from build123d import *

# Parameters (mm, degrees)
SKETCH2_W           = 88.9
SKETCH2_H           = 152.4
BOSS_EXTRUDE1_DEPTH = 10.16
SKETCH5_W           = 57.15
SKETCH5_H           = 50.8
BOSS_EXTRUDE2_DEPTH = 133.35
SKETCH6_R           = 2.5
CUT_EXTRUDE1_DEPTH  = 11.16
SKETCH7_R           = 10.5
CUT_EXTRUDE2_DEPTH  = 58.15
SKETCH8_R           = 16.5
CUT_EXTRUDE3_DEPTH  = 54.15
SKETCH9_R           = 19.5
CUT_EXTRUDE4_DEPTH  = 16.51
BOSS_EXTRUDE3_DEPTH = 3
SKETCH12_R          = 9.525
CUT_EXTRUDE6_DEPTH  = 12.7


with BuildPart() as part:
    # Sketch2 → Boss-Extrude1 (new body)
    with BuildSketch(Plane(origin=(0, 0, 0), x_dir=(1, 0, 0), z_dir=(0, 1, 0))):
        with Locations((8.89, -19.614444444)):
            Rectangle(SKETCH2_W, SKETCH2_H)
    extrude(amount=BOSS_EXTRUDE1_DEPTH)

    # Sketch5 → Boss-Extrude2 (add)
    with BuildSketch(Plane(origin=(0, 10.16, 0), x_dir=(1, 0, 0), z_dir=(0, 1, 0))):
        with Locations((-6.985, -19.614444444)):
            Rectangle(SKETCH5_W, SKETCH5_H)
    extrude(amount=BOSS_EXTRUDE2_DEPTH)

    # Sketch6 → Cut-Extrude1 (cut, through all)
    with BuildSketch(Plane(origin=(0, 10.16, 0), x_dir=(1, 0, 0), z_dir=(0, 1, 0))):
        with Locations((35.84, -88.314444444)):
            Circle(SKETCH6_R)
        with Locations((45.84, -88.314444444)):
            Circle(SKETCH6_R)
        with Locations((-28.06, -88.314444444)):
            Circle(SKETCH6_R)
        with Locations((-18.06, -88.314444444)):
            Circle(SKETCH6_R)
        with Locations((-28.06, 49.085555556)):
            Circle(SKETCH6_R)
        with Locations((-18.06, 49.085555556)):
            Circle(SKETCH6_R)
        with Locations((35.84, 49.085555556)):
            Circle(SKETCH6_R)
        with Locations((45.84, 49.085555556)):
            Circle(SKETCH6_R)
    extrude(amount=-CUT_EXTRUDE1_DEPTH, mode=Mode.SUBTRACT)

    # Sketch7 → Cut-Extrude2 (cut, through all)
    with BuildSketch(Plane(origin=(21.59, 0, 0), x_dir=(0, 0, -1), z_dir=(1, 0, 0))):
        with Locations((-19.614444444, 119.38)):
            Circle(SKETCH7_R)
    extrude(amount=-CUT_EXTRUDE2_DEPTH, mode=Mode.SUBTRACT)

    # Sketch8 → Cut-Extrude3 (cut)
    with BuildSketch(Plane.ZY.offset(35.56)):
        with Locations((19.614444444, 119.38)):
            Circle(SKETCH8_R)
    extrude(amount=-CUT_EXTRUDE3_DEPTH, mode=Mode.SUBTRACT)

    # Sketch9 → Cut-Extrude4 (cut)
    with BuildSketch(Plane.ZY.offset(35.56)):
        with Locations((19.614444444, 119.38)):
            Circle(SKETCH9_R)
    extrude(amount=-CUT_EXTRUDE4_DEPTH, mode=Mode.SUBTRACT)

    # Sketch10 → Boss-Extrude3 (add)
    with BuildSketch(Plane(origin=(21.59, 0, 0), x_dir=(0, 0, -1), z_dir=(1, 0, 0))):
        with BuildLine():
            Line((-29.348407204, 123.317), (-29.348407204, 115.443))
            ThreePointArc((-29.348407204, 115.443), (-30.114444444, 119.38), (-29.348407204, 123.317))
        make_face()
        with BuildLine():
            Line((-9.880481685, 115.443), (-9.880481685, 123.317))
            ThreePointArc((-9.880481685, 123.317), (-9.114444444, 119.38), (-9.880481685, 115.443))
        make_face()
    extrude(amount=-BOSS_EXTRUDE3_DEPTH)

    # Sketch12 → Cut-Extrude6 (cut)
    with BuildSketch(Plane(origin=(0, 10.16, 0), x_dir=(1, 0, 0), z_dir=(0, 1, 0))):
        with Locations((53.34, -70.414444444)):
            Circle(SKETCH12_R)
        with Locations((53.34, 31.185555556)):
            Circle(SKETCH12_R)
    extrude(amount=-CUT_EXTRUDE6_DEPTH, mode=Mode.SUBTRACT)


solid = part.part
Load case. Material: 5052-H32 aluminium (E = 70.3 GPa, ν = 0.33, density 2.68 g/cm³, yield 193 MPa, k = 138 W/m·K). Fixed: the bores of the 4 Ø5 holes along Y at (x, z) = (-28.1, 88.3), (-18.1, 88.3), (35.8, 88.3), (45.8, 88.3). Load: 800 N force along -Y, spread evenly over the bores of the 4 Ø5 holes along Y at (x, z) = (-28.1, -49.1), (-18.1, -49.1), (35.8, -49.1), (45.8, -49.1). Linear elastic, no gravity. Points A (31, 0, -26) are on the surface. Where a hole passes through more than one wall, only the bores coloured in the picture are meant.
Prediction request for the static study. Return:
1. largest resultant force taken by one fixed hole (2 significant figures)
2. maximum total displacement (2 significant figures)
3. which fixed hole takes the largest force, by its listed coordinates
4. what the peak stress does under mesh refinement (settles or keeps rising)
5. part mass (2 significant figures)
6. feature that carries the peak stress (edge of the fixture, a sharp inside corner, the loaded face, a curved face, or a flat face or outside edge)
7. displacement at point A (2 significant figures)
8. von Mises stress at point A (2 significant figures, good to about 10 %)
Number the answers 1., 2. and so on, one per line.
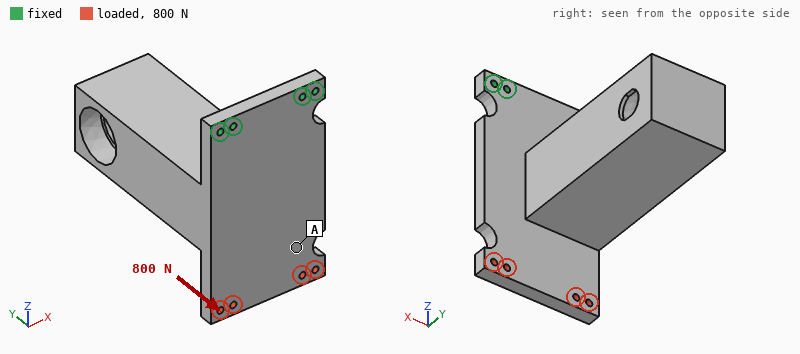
1. 390 N
2. 1.5 mm
3. (-18.1, 88.3)
4. keeps rising
5. 1.3 kg
6. edge of the fixture
7. 0.92 mm
8. 13 MPa
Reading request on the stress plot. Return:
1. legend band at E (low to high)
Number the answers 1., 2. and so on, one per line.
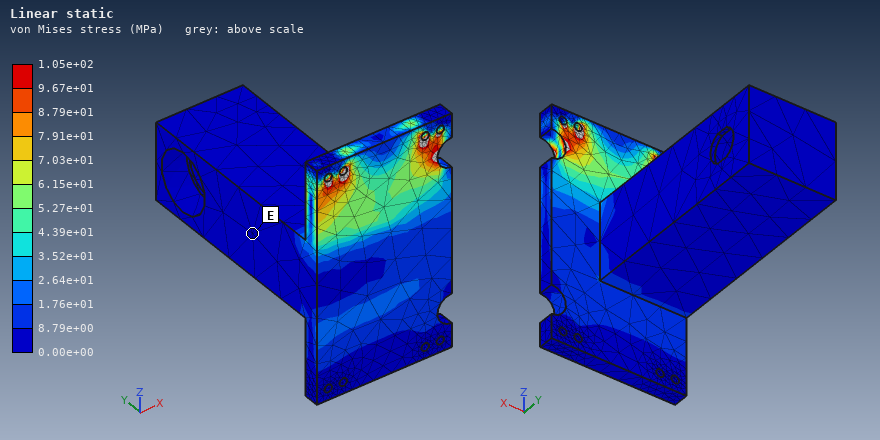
1. 0.00e+00 to 8.79e+00 MPa
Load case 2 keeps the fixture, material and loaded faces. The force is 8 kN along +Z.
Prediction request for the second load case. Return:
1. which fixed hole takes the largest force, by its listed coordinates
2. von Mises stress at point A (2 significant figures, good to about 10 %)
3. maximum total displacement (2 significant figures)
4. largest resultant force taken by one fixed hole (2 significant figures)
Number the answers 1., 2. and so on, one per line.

1. (35.8, 88.3)
2. 14 MPa
3. 44 µm
4. 3.1 kN
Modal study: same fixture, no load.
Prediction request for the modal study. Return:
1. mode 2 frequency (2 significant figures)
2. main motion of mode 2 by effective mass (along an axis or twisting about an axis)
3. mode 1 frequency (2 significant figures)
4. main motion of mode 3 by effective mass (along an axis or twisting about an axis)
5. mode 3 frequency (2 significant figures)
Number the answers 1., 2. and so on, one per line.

1. 390 Hz
2. along X
3. 170 Hz
4. along Y
5. 1100 Hz
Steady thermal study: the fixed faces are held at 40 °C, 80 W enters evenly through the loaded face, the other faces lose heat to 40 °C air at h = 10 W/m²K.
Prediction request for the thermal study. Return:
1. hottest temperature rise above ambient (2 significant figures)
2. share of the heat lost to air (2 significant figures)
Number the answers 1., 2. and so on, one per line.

1. 83 K
2. 27 %
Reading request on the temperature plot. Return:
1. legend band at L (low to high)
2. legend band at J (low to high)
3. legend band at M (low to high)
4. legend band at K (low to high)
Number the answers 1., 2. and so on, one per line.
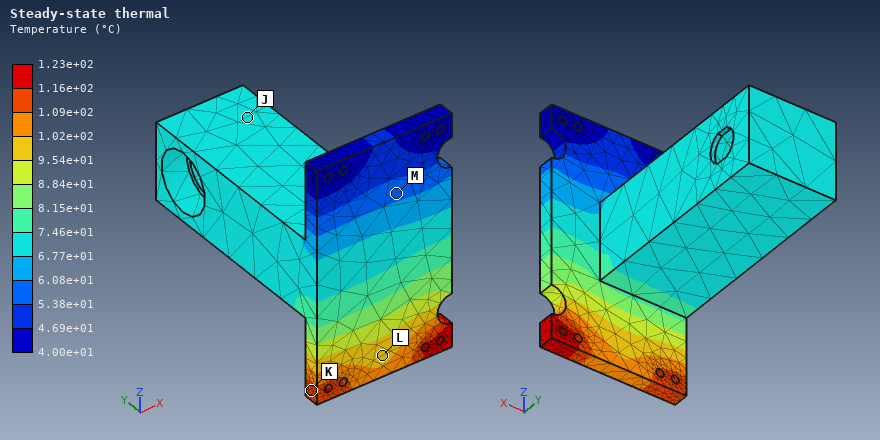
1. 9.54e+01 to 1.02e+02 °C
2. 6.77e+01 to 7.46e+01 °C
3. 5.38e+01 to 6.08e+01 °C
4. 1.09e+02 to 1.16e+02 °C
